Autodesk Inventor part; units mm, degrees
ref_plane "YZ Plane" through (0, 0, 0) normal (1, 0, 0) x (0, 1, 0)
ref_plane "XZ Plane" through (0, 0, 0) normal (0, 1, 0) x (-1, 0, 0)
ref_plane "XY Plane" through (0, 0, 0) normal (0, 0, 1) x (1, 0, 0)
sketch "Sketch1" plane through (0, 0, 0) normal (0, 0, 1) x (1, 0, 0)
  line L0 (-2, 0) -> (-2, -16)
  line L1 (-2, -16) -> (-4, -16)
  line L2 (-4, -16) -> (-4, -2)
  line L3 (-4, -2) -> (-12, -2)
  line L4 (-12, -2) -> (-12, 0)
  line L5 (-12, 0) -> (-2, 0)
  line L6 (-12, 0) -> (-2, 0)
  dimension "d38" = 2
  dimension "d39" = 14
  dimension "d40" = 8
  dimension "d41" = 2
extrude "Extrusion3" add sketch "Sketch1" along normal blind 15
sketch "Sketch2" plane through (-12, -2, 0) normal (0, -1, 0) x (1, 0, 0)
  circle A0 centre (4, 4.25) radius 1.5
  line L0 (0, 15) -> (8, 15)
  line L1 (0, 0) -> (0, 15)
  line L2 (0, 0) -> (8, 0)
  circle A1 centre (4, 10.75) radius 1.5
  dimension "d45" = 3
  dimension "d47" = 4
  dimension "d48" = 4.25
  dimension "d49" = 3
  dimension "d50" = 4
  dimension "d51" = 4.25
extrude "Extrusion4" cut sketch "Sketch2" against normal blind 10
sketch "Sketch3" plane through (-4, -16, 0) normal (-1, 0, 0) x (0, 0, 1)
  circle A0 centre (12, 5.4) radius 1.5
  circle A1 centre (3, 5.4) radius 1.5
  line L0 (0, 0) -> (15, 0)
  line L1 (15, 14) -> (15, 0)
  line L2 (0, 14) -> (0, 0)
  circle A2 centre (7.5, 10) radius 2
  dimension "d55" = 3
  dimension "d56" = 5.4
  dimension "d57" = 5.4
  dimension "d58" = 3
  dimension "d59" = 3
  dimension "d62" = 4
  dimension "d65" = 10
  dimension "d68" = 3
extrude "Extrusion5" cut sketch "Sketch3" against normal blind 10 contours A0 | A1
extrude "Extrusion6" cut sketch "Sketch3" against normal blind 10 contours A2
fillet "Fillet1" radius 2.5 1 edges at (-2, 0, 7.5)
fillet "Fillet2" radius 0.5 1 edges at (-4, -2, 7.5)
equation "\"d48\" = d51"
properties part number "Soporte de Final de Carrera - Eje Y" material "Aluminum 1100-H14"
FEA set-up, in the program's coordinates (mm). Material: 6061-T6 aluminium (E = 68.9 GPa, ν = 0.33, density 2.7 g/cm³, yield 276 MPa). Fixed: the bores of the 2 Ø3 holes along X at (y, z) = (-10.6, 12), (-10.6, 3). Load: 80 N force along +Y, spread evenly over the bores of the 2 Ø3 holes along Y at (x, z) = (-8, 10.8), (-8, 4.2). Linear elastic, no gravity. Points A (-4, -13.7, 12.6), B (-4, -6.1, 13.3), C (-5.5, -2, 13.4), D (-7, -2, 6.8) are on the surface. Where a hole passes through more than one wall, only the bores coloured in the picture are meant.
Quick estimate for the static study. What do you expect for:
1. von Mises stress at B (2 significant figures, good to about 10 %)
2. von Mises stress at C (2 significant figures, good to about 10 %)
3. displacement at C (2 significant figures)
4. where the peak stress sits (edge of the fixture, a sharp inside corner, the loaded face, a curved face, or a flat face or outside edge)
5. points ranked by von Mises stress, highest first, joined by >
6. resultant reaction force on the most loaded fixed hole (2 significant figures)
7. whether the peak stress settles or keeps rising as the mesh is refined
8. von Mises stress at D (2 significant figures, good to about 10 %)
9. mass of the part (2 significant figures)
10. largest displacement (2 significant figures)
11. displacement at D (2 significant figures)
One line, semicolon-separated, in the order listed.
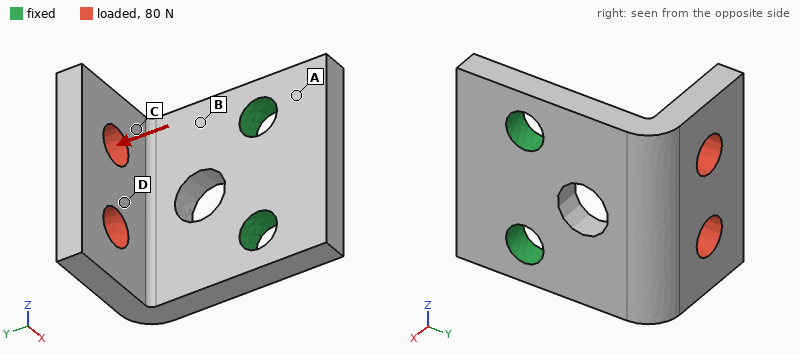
51 MPa; 20 MPa; 24 µm; a sharp inside corner; B > C > D > A; 41 N; keeps rising; 14 MPa; 1.7 g; 69 µm; 32 µm
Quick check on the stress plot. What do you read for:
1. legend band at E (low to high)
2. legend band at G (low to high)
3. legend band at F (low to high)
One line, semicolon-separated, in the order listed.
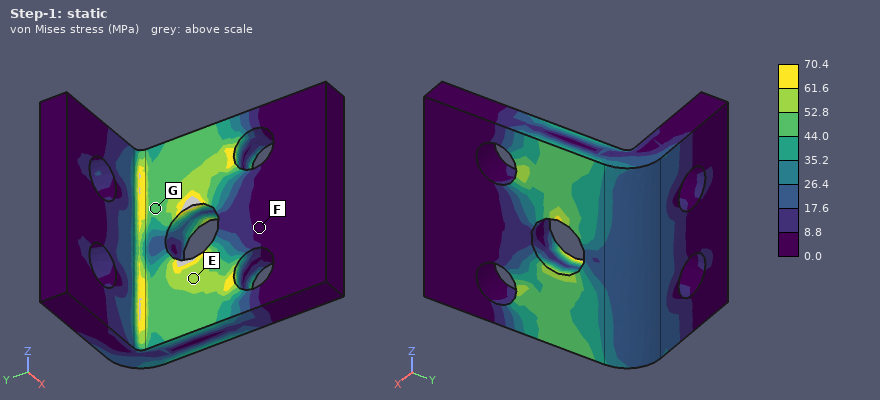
52.8 to 61.6 MPa; 44.0 to 52.8 MPa; 0.0 to 8.8 MPa
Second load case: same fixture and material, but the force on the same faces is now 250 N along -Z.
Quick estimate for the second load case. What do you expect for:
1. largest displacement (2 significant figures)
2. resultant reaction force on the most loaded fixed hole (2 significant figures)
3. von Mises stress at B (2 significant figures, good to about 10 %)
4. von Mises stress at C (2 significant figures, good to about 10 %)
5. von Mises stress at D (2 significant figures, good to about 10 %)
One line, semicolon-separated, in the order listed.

77 µm; 250 N; 79 MPa; 52 MPa; 41 MPa
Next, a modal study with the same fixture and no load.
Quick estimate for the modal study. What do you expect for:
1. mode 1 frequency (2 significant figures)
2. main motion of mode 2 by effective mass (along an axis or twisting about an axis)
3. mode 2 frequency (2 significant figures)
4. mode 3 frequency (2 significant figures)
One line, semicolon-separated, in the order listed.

6900 Hz; along Z; 12 kHz; 20 kHz
